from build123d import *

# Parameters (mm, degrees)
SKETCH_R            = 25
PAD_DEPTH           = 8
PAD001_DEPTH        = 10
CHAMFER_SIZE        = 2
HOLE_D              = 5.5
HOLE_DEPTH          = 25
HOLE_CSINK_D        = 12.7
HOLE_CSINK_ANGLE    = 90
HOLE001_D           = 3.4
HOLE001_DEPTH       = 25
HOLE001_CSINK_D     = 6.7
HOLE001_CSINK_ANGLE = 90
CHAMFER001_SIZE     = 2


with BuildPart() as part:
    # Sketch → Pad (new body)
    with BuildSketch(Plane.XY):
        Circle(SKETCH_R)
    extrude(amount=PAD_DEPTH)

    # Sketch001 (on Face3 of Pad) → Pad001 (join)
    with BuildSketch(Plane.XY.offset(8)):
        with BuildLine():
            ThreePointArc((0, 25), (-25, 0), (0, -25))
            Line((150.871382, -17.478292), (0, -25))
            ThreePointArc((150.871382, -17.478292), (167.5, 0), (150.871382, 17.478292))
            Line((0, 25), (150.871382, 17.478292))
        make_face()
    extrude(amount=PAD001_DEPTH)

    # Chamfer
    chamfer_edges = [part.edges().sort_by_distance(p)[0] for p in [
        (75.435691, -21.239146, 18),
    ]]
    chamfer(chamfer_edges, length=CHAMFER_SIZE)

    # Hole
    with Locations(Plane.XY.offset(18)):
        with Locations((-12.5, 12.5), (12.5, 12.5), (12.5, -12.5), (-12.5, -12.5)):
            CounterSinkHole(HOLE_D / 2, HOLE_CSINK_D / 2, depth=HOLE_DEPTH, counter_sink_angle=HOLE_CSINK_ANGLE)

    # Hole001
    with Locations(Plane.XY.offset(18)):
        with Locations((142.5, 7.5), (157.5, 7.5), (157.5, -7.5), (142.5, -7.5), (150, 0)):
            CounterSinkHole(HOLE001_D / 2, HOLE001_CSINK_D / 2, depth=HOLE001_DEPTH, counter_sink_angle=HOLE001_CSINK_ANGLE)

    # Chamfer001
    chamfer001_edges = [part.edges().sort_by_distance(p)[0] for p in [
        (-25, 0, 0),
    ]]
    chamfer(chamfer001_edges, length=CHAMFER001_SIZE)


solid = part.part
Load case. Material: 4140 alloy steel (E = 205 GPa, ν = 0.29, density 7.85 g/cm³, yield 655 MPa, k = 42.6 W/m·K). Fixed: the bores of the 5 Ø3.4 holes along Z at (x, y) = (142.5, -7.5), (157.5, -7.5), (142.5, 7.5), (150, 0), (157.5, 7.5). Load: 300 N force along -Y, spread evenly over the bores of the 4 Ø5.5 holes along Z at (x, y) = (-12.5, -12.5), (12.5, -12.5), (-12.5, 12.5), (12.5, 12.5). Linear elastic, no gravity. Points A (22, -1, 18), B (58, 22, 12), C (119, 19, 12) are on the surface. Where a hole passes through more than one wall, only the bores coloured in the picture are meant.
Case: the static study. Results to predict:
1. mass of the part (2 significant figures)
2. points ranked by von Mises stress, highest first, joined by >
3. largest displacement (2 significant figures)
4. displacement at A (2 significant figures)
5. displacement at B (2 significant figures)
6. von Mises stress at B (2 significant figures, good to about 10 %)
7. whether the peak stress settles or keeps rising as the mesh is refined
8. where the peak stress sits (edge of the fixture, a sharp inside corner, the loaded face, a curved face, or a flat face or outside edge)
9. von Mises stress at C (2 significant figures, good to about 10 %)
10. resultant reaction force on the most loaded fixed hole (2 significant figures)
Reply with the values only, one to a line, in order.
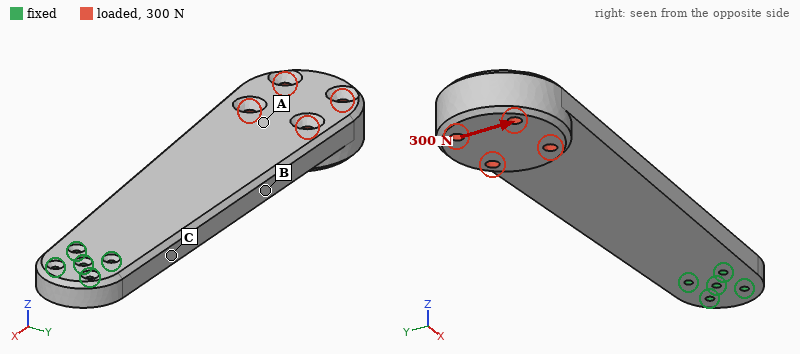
710 g
C > B > A
48 µm
29 µm
20 µm
5.5 MPa
keeps rising
edge of the fixture
15 MPa
1.6 kN
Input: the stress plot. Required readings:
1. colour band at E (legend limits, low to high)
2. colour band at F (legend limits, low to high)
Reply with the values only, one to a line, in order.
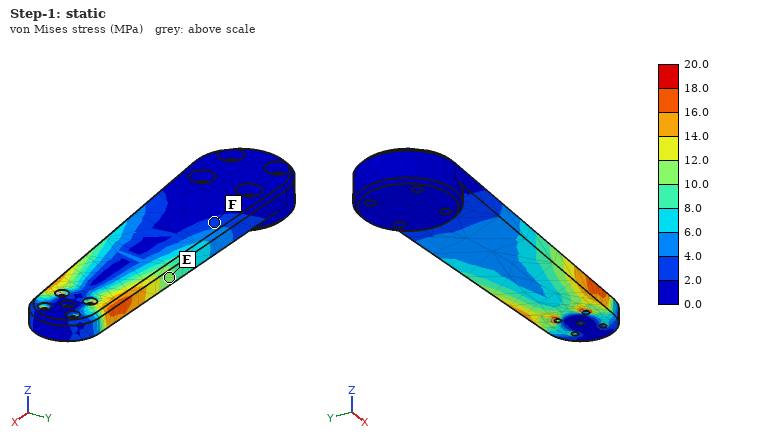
10.0 to 12.0 MPa
2.0 to 4.0 MPa
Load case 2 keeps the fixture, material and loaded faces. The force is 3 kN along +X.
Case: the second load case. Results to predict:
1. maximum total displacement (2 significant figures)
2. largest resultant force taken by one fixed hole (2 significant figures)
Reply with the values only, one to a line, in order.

0.34 mm
1.2 kN
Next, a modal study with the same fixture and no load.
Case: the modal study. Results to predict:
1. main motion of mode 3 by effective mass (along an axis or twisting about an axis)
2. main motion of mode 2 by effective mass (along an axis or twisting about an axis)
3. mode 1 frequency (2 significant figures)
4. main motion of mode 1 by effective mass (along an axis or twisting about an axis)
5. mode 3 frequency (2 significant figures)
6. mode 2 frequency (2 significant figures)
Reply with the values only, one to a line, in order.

twisting about X
along Y
220 Hz
along Z
1600 Hz
770 Hz
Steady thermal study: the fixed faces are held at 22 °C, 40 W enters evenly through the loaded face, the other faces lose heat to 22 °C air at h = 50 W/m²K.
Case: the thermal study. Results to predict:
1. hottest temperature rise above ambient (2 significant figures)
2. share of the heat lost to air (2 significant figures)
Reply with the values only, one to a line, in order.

75 K
89 %
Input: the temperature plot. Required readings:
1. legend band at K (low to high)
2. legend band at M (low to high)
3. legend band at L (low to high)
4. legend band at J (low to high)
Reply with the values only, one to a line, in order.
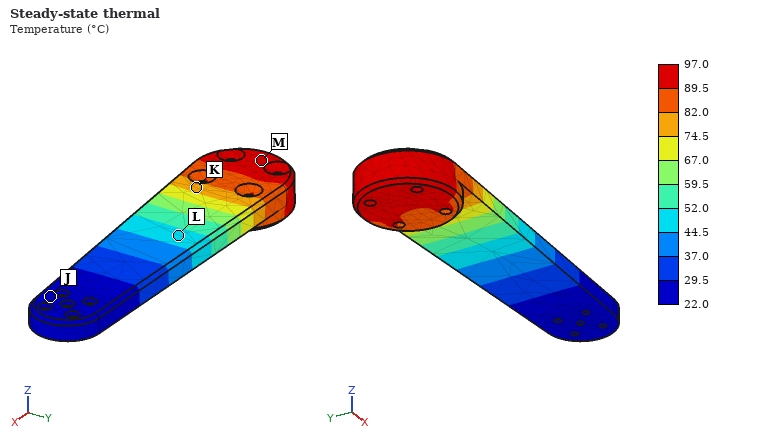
74.5 to 82.0 °C
89.5 to 97.0 °C
44.5 to 52.0 °C
22.0 to 29.5 °C
